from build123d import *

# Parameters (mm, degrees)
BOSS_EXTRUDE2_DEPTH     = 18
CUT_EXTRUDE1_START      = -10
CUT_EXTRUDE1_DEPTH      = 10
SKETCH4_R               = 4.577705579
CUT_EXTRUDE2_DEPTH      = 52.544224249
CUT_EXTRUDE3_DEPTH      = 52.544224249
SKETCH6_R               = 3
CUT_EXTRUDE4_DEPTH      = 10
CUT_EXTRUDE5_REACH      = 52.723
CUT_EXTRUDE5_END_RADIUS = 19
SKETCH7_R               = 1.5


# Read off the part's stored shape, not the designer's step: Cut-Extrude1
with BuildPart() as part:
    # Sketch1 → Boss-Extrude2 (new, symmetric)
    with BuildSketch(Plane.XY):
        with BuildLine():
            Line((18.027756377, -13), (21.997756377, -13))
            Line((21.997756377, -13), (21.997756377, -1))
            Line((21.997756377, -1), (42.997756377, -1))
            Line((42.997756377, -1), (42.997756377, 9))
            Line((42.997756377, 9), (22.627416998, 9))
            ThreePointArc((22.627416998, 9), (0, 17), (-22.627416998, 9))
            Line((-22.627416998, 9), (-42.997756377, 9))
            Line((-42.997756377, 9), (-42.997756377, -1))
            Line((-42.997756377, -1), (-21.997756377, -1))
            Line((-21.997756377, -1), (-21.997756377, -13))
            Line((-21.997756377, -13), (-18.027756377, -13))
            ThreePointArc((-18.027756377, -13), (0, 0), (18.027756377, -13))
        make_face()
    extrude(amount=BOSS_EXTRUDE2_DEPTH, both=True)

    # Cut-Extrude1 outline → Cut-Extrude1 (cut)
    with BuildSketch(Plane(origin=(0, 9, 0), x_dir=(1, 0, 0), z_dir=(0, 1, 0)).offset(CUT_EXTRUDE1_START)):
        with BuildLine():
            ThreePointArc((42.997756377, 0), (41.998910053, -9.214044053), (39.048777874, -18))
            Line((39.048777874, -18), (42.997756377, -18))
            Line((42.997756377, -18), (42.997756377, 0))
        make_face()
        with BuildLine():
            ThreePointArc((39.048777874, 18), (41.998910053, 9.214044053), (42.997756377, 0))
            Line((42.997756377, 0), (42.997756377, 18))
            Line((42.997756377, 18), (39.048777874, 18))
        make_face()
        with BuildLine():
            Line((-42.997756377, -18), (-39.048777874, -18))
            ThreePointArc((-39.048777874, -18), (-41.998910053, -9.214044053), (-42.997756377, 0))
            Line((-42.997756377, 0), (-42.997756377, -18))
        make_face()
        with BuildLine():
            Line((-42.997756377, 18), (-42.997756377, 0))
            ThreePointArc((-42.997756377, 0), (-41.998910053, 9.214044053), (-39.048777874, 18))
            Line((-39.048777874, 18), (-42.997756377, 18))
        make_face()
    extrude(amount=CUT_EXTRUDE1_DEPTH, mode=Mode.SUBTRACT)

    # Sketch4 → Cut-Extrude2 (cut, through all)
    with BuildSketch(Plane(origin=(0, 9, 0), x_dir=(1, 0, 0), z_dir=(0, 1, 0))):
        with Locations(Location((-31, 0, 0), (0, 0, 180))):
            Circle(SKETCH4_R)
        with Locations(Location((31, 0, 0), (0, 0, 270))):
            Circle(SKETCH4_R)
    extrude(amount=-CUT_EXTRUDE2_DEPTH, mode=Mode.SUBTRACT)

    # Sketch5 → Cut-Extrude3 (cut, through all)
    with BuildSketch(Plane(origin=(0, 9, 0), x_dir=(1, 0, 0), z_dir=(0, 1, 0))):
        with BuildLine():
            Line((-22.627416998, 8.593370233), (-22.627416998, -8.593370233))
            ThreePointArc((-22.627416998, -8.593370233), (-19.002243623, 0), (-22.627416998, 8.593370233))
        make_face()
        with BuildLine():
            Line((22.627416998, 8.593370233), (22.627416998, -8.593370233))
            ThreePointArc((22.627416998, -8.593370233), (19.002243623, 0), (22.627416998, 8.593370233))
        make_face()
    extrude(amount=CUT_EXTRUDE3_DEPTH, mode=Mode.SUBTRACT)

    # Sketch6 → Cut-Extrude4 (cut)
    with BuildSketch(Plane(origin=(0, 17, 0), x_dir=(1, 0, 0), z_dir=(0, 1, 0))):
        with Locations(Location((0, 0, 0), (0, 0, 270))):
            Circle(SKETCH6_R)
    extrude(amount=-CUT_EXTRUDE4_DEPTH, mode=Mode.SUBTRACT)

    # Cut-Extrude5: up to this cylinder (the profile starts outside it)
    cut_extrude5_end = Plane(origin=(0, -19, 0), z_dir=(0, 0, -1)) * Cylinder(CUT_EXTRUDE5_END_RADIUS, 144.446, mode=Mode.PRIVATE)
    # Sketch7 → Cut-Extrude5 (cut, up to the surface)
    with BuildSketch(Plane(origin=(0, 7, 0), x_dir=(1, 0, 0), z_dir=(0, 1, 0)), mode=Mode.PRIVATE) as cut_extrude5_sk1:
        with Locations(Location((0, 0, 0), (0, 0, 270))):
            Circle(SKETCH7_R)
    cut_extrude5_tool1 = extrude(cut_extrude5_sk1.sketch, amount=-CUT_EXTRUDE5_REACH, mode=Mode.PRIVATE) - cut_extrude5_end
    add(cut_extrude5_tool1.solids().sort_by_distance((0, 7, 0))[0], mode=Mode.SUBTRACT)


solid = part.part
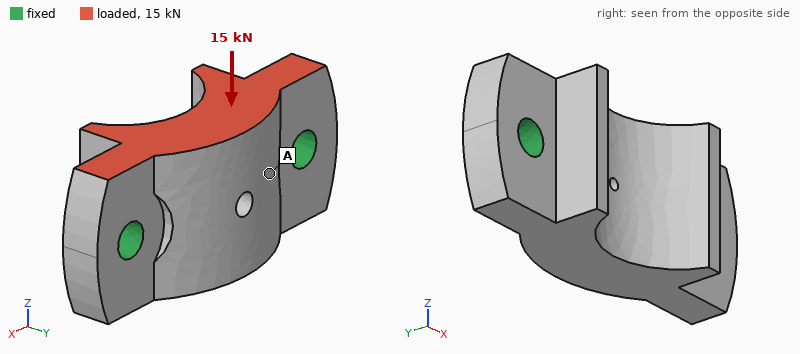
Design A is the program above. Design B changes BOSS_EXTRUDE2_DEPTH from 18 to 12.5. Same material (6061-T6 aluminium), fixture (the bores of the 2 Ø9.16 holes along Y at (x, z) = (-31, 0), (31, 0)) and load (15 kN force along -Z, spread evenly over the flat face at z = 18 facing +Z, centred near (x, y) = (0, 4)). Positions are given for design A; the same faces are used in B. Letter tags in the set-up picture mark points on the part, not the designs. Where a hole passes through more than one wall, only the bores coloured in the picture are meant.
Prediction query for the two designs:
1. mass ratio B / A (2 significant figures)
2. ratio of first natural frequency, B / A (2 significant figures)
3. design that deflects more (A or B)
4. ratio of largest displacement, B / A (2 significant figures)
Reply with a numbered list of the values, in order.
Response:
1. 0.69
2. 1.3
3. B
4. 1.4
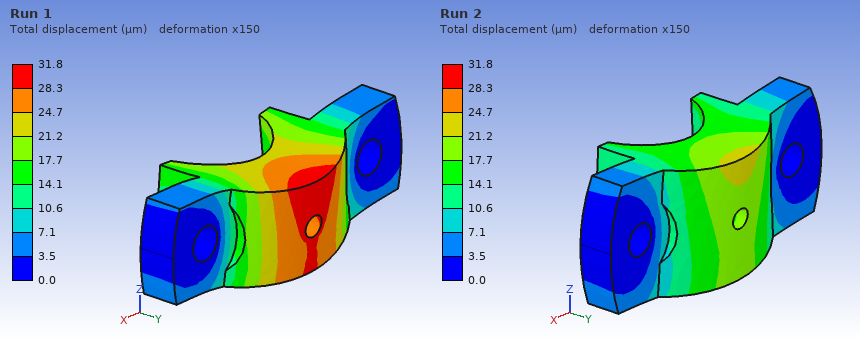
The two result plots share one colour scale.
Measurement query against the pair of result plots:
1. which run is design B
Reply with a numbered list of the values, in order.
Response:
1. Run 1
